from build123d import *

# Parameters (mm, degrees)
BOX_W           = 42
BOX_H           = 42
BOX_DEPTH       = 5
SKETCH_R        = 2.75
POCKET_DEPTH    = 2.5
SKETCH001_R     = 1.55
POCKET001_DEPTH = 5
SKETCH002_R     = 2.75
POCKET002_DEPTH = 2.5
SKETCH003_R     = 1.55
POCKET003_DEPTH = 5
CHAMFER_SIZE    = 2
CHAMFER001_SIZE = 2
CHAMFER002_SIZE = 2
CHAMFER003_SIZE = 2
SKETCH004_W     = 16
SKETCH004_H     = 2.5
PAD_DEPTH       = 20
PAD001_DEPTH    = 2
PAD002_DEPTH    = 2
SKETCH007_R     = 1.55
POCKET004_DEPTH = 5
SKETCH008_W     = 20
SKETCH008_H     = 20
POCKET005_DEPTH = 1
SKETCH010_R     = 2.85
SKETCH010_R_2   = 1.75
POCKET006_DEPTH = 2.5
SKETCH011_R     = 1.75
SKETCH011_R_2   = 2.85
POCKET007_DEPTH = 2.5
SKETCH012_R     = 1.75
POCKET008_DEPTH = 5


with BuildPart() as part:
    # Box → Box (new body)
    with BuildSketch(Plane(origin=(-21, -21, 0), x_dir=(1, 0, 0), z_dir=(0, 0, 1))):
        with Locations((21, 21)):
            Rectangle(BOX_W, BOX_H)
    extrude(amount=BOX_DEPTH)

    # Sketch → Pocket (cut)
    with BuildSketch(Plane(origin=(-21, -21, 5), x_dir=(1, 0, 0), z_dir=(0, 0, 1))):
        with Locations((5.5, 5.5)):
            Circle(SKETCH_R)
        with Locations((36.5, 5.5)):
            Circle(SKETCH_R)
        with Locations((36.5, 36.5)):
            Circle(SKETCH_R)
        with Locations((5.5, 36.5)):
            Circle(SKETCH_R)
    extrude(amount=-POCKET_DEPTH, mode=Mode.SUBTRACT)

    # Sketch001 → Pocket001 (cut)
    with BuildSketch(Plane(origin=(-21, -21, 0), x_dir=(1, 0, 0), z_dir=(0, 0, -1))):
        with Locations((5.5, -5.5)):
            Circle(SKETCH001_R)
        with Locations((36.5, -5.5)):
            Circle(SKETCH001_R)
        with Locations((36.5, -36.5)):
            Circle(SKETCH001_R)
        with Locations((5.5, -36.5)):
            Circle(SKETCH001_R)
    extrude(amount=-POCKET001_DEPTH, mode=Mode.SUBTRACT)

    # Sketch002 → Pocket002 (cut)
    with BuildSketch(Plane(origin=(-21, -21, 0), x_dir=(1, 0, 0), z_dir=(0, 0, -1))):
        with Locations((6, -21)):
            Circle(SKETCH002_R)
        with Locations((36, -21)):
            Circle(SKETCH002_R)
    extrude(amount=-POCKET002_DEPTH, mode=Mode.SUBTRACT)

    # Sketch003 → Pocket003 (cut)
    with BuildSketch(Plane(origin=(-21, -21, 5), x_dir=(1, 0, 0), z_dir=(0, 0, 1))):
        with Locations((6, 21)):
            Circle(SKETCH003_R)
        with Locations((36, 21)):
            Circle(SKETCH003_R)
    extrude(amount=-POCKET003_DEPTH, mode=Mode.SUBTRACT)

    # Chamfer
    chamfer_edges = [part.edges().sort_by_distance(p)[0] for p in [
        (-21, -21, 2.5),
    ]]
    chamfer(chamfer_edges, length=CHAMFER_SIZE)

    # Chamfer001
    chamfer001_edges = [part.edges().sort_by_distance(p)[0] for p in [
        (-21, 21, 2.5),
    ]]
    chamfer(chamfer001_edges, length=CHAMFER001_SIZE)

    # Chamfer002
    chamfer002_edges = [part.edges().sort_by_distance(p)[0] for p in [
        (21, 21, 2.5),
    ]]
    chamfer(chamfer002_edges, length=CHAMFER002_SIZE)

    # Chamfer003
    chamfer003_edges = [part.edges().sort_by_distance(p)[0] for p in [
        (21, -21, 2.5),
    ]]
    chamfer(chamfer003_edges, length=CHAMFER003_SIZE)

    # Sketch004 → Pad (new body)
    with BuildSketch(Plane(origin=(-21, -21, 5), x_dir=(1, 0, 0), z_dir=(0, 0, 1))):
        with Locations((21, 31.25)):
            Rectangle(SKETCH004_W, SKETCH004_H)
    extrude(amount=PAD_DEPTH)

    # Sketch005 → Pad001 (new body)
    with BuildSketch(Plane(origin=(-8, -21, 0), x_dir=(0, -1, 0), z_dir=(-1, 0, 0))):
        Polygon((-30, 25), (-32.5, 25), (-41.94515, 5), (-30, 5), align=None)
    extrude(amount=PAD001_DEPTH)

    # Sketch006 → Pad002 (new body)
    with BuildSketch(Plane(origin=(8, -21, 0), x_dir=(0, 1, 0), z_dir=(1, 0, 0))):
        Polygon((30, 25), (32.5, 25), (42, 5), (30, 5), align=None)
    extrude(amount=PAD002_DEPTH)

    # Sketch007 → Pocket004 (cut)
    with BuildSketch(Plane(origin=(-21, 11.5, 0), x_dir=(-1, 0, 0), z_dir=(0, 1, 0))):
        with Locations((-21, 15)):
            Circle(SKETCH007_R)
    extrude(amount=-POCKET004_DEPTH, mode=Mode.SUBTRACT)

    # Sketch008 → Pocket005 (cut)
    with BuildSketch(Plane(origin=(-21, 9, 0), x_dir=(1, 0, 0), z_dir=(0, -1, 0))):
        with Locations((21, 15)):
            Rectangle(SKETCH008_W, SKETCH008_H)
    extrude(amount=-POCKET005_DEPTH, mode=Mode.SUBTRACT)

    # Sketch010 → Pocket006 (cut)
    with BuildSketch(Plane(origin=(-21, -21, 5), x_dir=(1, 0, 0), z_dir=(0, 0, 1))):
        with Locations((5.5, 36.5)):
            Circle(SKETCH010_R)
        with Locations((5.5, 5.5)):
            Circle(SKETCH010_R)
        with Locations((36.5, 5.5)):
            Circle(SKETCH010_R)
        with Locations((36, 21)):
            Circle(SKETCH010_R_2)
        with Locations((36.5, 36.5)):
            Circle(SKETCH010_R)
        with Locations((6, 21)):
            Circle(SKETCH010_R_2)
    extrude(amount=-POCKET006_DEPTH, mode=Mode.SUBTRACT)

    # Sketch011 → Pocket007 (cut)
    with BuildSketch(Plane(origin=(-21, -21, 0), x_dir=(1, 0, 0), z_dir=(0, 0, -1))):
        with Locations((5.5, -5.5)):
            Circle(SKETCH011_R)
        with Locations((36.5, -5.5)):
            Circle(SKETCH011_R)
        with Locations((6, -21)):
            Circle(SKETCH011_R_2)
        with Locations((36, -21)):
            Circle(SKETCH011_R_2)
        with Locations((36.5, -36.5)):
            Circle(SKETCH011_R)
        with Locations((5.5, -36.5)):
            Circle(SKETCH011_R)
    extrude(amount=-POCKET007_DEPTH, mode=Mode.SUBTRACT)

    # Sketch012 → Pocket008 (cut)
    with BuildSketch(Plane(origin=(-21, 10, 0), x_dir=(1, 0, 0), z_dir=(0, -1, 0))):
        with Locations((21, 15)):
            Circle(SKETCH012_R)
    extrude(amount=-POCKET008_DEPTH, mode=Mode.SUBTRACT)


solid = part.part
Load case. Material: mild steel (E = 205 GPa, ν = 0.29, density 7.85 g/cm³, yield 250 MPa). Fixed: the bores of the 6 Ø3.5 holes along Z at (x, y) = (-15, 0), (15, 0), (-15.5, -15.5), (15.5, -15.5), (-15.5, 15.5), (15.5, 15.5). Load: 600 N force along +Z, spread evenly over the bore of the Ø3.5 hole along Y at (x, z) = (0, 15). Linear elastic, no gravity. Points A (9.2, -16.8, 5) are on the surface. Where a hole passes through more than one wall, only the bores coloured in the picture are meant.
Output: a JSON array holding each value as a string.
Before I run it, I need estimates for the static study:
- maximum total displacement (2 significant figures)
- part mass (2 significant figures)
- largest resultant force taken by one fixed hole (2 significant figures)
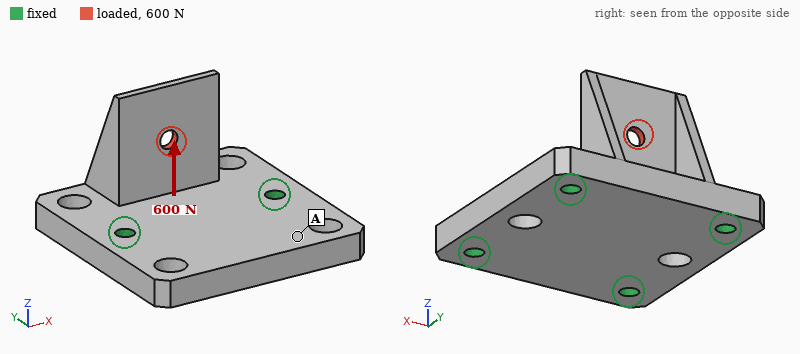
["5.0 µm", "72 g", "250 N"]
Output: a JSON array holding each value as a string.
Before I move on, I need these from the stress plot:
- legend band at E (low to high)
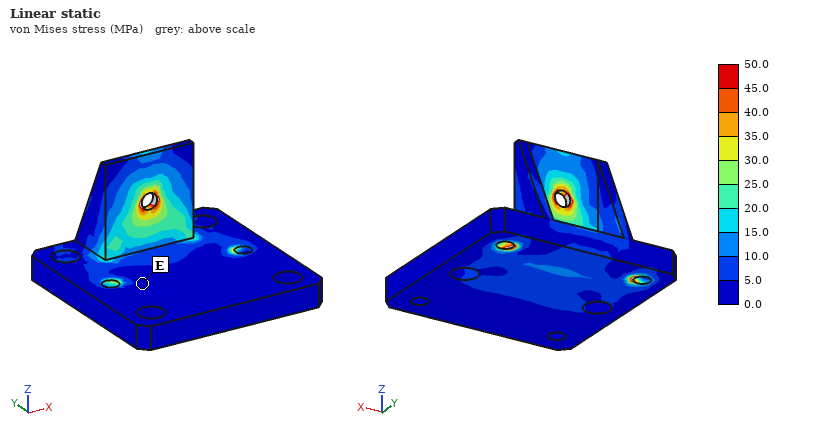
["0.0 to 5.0 MPa"]
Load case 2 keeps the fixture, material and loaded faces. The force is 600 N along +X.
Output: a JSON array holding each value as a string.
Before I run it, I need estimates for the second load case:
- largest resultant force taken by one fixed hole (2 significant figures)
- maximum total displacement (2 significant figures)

["310 N", "8.2 µm"]
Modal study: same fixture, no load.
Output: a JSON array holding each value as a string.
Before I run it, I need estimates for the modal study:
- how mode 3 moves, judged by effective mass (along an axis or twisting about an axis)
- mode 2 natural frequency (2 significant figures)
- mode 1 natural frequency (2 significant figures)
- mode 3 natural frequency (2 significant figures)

["along Z", "16 kHz", "11 kHz", "19 kHz"]
